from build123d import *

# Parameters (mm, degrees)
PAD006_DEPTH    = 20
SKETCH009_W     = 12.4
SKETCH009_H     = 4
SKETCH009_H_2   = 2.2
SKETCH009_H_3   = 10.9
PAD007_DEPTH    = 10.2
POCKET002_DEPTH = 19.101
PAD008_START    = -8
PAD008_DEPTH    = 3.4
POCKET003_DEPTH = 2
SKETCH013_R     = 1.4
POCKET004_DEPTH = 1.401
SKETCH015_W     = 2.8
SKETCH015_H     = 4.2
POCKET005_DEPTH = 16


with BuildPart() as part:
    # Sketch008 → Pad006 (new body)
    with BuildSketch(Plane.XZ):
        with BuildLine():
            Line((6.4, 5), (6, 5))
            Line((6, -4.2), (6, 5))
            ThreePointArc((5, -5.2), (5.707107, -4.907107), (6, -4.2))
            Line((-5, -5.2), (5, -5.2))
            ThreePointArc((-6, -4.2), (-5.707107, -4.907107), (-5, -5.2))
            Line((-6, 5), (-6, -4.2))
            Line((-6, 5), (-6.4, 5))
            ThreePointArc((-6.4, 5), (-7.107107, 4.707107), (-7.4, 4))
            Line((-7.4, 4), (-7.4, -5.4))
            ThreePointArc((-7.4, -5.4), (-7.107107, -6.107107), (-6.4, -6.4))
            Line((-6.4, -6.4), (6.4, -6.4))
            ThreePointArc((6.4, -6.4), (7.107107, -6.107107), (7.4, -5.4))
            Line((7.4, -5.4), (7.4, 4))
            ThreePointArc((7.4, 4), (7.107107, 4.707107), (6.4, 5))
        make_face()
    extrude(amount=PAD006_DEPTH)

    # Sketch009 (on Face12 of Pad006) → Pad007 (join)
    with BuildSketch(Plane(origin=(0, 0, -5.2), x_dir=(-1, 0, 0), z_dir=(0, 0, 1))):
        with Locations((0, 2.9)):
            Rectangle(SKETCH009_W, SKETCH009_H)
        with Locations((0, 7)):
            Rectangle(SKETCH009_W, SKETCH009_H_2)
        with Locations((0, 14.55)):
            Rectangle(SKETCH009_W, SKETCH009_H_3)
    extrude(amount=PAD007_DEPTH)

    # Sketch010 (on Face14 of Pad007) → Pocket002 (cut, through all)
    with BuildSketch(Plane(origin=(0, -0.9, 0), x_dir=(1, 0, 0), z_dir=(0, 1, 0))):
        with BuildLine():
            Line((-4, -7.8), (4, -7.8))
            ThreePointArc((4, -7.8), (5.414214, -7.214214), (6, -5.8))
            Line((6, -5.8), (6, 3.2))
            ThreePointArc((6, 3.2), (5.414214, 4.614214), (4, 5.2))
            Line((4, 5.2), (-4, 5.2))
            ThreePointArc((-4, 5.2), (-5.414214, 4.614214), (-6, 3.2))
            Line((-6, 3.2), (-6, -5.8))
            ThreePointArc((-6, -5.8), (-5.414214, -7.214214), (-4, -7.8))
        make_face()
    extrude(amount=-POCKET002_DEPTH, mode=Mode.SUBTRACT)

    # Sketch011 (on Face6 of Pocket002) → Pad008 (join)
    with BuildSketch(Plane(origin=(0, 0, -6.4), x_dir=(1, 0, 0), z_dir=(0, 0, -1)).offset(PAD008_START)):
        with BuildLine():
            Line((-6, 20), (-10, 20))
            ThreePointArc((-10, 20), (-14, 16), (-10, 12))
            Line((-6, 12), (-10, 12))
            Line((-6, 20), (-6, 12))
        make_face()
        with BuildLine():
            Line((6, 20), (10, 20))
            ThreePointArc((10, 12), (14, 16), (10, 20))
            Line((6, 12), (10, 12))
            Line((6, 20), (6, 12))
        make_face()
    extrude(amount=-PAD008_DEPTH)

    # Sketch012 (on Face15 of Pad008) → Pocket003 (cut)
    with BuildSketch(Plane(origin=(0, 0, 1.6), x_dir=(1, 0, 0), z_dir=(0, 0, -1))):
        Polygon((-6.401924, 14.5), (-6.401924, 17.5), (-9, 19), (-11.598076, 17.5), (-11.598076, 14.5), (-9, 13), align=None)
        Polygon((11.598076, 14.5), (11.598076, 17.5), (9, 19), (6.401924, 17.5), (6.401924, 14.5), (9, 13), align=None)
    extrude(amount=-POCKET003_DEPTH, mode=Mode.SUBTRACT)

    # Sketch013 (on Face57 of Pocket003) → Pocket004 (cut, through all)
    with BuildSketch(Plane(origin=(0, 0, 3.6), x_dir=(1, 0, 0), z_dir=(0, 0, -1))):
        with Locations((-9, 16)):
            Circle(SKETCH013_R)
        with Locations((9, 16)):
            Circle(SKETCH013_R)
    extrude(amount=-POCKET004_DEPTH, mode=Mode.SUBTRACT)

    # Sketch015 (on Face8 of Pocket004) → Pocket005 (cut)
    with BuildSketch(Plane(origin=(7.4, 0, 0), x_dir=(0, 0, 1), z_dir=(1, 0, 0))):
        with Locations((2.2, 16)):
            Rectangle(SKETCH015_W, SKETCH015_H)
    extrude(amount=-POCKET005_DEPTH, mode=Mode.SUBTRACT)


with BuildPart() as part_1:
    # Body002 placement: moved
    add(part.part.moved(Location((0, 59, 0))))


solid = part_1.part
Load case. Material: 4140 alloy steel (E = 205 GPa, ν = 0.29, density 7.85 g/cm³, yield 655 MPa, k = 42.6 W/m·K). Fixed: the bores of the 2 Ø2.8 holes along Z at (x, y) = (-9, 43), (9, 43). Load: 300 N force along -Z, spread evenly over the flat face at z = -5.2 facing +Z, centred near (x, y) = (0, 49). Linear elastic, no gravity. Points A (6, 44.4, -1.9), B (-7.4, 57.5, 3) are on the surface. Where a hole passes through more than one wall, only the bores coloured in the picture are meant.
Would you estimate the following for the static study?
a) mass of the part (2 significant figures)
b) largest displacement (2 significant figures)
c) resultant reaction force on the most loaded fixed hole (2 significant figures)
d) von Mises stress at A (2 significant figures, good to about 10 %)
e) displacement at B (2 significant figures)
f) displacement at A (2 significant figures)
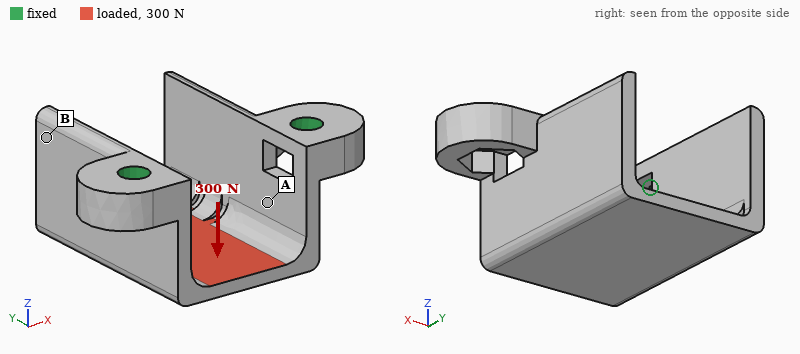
8.8 g
35 µm
160 N
51 MPa
22 µm
9.3 µm
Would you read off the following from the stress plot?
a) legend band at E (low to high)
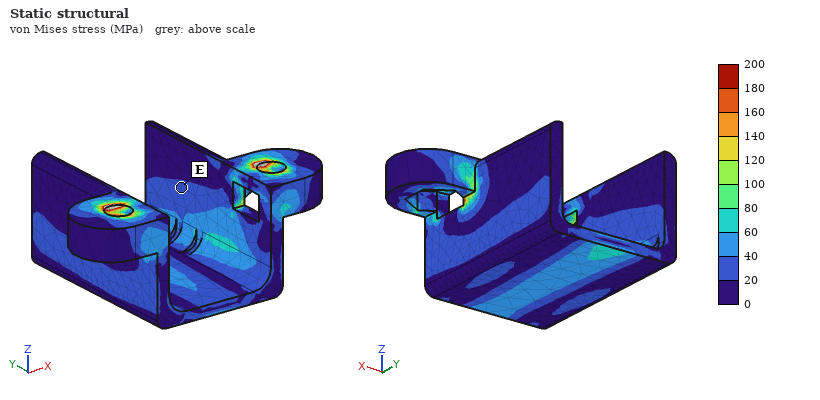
20 to 40 MPa
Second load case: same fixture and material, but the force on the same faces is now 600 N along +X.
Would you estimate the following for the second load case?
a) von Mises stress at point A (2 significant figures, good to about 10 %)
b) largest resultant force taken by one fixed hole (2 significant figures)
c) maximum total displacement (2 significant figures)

76 MPa
400 N
66 µm
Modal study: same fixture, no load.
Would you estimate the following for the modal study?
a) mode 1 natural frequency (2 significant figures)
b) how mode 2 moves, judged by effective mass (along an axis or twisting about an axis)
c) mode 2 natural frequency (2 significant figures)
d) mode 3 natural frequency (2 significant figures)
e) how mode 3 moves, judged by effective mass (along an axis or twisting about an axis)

5900 Hz
along X
6600 Hz
9900 Hz
along X
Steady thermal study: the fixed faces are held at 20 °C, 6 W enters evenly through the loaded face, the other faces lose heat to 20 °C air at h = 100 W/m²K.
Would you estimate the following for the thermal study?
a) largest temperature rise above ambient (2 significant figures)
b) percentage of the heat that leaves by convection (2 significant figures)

40 K
54 %
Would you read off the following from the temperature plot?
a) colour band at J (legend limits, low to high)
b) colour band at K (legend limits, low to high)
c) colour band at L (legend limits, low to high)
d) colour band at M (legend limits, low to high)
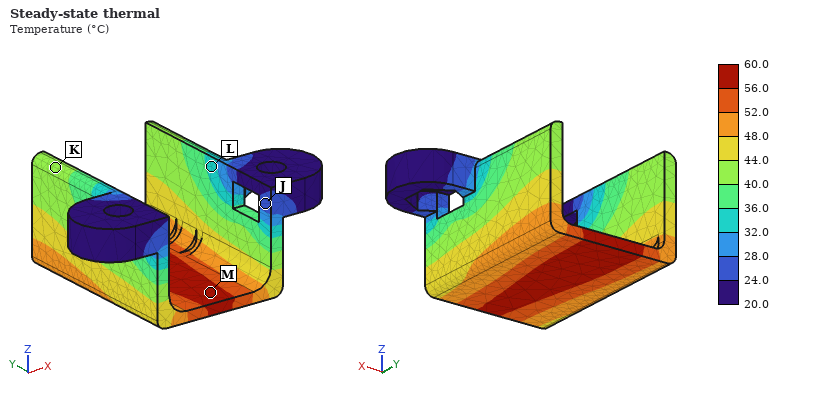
24.0 to 28.0 °C
40.0 to 44.0 °C
32.0 to 36.0 °C
56.0 to 60.0 °C
